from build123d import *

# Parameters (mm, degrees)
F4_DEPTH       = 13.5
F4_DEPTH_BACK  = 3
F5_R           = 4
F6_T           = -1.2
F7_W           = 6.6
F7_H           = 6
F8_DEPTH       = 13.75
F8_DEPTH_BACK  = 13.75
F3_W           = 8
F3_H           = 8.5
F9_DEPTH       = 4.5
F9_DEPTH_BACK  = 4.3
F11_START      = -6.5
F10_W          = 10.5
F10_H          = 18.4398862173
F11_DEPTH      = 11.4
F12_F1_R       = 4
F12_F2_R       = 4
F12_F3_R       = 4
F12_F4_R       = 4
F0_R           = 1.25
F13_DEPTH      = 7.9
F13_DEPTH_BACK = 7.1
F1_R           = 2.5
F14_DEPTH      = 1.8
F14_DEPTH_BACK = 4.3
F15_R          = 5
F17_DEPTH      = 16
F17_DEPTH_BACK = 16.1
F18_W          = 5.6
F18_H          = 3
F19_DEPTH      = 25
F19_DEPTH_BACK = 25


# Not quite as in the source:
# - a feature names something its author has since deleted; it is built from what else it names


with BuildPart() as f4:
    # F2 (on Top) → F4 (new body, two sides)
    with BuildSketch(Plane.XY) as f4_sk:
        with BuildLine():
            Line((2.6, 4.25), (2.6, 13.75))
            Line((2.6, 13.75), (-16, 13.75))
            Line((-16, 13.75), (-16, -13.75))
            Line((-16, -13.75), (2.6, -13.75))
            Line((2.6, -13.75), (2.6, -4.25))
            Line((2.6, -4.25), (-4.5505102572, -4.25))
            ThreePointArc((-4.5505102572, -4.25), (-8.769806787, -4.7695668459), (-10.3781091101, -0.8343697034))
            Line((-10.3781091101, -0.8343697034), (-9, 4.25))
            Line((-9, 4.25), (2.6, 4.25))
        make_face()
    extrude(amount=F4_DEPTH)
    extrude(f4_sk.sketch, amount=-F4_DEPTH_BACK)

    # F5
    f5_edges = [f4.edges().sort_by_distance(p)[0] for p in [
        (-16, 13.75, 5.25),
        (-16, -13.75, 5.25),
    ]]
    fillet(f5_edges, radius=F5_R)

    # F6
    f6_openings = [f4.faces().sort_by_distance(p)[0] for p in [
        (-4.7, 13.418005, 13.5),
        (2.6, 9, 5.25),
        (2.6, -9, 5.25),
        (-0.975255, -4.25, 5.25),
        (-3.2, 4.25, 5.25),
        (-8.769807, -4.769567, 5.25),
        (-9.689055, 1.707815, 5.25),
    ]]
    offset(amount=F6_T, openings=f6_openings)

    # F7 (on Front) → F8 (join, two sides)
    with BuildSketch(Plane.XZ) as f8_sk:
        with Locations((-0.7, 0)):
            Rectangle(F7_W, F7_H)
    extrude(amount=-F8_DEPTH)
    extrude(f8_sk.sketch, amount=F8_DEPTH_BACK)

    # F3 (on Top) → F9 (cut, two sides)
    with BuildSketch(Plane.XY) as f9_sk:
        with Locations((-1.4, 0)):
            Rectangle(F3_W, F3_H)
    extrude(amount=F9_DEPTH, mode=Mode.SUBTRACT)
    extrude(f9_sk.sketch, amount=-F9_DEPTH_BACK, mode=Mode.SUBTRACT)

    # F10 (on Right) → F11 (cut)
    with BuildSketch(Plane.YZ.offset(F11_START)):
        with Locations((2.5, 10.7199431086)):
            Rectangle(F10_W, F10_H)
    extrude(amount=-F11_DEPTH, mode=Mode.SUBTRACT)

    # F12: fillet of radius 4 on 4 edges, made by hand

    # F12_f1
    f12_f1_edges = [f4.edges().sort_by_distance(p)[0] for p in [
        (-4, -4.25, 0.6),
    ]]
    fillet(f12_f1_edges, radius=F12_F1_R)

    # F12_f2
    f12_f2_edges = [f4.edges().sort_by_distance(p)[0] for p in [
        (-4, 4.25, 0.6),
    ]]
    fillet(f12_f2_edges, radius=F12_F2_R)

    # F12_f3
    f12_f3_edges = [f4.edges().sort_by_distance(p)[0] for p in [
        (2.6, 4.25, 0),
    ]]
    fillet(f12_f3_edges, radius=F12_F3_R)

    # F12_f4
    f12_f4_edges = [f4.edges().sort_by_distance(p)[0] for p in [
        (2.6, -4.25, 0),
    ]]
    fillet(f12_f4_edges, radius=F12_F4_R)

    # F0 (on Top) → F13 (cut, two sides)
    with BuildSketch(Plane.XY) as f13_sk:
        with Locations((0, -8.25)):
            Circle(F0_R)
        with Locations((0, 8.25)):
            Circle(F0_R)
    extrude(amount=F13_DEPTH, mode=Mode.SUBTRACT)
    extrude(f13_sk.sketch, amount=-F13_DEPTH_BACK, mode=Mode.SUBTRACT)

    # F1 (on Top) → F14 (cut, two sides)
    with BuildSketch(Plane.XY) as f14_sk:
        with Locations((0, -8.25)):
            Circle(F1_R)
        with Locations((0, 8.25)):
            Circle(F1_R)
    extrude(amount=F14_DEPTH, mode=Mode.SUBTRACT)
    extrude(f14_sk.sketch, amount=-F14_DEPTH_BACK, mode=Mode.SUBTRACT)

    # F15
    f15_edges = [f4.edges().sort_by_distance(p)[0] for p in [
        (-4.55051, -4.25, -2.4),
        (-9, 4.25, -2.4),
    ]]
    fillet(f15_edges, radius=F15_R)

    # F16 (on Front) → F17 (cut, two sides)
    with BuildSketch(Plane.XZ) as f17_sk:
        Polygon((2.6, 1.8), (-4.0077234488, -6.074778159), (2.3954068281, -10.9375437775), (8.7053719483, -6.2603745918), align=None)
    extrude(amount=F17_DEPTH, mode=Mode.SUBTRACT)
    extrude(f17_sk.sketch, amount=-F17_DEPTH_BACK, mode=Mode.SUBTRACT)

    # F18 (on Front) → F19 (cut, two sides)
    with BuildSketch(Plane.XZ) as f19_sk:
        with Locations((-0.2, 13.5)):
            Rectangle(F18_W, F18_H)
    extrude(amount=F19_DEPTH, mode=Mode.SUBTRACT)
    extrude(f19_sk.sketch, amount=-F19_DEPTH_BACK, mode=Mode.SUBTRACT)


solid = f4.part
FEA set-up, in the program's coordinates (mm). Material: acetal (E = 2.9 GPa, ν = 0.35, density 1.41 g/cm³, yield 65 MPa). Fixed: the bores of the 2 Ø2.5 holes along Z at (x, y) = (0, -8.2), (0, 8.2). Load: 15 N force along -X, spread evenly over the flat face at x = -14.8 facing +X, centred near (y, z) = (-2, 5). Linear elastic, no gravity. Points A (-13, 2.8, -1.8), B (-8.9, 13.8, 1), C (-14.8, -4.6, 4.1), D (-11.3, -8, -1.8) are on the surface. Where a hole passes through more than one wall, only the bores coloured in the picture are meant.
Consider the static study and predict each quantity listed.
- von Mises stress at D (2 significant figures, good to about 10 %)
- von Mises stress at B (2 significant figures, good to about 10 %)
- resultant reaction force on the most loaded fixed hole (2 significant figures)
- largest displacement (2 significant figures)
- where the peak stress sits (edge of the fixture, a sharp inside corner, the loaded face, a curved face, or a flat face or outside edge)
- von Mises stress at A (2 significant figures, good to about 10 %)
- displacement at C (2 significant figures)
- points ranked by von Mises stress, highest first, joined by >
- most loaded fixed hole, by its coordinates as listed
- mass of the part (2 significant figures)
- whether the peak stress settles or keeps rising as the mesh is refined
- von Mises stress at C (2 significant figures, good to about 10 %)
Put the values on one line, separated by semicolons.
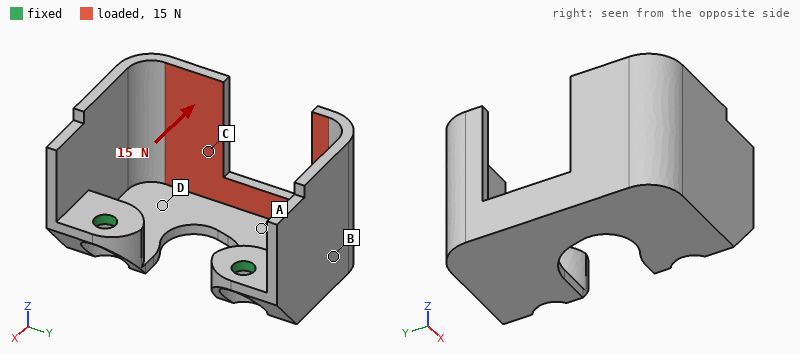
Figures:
2.3 MPa; 0.91 MPa; 9.3 N; 0.43 mm; edge of the fixture; 3.5 MPa; 0.16 mm; C > A > D > B; (0, -8.2); 2.2 g; keeps rising; 6.3 MPa
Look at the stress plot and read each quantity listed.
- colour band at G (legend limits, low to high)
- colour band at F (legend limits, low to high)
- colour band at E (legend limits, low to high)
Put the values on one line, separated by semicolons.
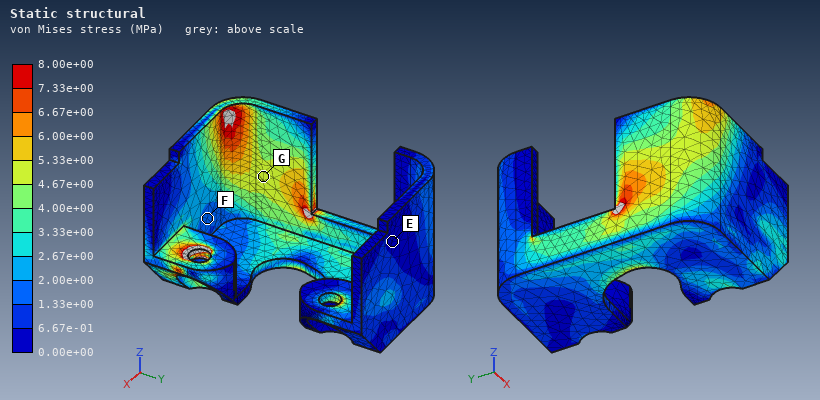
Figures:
4.67e+00 to 5.33e+00 MPa; 1.33e+00 to 2.00e+00 MPa; 0.00e+00 to 6.67e-01 MPa
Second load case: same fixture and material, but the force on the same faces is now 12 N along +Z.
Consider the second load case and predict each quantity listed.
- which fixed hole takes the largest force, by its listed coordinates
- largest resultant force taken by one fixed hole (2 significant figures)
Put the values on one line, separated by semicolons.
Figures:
(0, -8.2); 6.7 N
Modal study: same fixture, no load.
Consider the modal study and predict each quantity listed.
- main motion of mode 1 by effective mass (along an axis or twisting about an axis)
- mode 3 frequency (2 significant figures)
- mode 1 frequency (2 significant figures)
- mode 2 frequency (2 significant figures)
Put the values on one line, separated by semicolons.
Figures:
along Z; 2200 Hz; 1000 Hz; 1100 Hz
